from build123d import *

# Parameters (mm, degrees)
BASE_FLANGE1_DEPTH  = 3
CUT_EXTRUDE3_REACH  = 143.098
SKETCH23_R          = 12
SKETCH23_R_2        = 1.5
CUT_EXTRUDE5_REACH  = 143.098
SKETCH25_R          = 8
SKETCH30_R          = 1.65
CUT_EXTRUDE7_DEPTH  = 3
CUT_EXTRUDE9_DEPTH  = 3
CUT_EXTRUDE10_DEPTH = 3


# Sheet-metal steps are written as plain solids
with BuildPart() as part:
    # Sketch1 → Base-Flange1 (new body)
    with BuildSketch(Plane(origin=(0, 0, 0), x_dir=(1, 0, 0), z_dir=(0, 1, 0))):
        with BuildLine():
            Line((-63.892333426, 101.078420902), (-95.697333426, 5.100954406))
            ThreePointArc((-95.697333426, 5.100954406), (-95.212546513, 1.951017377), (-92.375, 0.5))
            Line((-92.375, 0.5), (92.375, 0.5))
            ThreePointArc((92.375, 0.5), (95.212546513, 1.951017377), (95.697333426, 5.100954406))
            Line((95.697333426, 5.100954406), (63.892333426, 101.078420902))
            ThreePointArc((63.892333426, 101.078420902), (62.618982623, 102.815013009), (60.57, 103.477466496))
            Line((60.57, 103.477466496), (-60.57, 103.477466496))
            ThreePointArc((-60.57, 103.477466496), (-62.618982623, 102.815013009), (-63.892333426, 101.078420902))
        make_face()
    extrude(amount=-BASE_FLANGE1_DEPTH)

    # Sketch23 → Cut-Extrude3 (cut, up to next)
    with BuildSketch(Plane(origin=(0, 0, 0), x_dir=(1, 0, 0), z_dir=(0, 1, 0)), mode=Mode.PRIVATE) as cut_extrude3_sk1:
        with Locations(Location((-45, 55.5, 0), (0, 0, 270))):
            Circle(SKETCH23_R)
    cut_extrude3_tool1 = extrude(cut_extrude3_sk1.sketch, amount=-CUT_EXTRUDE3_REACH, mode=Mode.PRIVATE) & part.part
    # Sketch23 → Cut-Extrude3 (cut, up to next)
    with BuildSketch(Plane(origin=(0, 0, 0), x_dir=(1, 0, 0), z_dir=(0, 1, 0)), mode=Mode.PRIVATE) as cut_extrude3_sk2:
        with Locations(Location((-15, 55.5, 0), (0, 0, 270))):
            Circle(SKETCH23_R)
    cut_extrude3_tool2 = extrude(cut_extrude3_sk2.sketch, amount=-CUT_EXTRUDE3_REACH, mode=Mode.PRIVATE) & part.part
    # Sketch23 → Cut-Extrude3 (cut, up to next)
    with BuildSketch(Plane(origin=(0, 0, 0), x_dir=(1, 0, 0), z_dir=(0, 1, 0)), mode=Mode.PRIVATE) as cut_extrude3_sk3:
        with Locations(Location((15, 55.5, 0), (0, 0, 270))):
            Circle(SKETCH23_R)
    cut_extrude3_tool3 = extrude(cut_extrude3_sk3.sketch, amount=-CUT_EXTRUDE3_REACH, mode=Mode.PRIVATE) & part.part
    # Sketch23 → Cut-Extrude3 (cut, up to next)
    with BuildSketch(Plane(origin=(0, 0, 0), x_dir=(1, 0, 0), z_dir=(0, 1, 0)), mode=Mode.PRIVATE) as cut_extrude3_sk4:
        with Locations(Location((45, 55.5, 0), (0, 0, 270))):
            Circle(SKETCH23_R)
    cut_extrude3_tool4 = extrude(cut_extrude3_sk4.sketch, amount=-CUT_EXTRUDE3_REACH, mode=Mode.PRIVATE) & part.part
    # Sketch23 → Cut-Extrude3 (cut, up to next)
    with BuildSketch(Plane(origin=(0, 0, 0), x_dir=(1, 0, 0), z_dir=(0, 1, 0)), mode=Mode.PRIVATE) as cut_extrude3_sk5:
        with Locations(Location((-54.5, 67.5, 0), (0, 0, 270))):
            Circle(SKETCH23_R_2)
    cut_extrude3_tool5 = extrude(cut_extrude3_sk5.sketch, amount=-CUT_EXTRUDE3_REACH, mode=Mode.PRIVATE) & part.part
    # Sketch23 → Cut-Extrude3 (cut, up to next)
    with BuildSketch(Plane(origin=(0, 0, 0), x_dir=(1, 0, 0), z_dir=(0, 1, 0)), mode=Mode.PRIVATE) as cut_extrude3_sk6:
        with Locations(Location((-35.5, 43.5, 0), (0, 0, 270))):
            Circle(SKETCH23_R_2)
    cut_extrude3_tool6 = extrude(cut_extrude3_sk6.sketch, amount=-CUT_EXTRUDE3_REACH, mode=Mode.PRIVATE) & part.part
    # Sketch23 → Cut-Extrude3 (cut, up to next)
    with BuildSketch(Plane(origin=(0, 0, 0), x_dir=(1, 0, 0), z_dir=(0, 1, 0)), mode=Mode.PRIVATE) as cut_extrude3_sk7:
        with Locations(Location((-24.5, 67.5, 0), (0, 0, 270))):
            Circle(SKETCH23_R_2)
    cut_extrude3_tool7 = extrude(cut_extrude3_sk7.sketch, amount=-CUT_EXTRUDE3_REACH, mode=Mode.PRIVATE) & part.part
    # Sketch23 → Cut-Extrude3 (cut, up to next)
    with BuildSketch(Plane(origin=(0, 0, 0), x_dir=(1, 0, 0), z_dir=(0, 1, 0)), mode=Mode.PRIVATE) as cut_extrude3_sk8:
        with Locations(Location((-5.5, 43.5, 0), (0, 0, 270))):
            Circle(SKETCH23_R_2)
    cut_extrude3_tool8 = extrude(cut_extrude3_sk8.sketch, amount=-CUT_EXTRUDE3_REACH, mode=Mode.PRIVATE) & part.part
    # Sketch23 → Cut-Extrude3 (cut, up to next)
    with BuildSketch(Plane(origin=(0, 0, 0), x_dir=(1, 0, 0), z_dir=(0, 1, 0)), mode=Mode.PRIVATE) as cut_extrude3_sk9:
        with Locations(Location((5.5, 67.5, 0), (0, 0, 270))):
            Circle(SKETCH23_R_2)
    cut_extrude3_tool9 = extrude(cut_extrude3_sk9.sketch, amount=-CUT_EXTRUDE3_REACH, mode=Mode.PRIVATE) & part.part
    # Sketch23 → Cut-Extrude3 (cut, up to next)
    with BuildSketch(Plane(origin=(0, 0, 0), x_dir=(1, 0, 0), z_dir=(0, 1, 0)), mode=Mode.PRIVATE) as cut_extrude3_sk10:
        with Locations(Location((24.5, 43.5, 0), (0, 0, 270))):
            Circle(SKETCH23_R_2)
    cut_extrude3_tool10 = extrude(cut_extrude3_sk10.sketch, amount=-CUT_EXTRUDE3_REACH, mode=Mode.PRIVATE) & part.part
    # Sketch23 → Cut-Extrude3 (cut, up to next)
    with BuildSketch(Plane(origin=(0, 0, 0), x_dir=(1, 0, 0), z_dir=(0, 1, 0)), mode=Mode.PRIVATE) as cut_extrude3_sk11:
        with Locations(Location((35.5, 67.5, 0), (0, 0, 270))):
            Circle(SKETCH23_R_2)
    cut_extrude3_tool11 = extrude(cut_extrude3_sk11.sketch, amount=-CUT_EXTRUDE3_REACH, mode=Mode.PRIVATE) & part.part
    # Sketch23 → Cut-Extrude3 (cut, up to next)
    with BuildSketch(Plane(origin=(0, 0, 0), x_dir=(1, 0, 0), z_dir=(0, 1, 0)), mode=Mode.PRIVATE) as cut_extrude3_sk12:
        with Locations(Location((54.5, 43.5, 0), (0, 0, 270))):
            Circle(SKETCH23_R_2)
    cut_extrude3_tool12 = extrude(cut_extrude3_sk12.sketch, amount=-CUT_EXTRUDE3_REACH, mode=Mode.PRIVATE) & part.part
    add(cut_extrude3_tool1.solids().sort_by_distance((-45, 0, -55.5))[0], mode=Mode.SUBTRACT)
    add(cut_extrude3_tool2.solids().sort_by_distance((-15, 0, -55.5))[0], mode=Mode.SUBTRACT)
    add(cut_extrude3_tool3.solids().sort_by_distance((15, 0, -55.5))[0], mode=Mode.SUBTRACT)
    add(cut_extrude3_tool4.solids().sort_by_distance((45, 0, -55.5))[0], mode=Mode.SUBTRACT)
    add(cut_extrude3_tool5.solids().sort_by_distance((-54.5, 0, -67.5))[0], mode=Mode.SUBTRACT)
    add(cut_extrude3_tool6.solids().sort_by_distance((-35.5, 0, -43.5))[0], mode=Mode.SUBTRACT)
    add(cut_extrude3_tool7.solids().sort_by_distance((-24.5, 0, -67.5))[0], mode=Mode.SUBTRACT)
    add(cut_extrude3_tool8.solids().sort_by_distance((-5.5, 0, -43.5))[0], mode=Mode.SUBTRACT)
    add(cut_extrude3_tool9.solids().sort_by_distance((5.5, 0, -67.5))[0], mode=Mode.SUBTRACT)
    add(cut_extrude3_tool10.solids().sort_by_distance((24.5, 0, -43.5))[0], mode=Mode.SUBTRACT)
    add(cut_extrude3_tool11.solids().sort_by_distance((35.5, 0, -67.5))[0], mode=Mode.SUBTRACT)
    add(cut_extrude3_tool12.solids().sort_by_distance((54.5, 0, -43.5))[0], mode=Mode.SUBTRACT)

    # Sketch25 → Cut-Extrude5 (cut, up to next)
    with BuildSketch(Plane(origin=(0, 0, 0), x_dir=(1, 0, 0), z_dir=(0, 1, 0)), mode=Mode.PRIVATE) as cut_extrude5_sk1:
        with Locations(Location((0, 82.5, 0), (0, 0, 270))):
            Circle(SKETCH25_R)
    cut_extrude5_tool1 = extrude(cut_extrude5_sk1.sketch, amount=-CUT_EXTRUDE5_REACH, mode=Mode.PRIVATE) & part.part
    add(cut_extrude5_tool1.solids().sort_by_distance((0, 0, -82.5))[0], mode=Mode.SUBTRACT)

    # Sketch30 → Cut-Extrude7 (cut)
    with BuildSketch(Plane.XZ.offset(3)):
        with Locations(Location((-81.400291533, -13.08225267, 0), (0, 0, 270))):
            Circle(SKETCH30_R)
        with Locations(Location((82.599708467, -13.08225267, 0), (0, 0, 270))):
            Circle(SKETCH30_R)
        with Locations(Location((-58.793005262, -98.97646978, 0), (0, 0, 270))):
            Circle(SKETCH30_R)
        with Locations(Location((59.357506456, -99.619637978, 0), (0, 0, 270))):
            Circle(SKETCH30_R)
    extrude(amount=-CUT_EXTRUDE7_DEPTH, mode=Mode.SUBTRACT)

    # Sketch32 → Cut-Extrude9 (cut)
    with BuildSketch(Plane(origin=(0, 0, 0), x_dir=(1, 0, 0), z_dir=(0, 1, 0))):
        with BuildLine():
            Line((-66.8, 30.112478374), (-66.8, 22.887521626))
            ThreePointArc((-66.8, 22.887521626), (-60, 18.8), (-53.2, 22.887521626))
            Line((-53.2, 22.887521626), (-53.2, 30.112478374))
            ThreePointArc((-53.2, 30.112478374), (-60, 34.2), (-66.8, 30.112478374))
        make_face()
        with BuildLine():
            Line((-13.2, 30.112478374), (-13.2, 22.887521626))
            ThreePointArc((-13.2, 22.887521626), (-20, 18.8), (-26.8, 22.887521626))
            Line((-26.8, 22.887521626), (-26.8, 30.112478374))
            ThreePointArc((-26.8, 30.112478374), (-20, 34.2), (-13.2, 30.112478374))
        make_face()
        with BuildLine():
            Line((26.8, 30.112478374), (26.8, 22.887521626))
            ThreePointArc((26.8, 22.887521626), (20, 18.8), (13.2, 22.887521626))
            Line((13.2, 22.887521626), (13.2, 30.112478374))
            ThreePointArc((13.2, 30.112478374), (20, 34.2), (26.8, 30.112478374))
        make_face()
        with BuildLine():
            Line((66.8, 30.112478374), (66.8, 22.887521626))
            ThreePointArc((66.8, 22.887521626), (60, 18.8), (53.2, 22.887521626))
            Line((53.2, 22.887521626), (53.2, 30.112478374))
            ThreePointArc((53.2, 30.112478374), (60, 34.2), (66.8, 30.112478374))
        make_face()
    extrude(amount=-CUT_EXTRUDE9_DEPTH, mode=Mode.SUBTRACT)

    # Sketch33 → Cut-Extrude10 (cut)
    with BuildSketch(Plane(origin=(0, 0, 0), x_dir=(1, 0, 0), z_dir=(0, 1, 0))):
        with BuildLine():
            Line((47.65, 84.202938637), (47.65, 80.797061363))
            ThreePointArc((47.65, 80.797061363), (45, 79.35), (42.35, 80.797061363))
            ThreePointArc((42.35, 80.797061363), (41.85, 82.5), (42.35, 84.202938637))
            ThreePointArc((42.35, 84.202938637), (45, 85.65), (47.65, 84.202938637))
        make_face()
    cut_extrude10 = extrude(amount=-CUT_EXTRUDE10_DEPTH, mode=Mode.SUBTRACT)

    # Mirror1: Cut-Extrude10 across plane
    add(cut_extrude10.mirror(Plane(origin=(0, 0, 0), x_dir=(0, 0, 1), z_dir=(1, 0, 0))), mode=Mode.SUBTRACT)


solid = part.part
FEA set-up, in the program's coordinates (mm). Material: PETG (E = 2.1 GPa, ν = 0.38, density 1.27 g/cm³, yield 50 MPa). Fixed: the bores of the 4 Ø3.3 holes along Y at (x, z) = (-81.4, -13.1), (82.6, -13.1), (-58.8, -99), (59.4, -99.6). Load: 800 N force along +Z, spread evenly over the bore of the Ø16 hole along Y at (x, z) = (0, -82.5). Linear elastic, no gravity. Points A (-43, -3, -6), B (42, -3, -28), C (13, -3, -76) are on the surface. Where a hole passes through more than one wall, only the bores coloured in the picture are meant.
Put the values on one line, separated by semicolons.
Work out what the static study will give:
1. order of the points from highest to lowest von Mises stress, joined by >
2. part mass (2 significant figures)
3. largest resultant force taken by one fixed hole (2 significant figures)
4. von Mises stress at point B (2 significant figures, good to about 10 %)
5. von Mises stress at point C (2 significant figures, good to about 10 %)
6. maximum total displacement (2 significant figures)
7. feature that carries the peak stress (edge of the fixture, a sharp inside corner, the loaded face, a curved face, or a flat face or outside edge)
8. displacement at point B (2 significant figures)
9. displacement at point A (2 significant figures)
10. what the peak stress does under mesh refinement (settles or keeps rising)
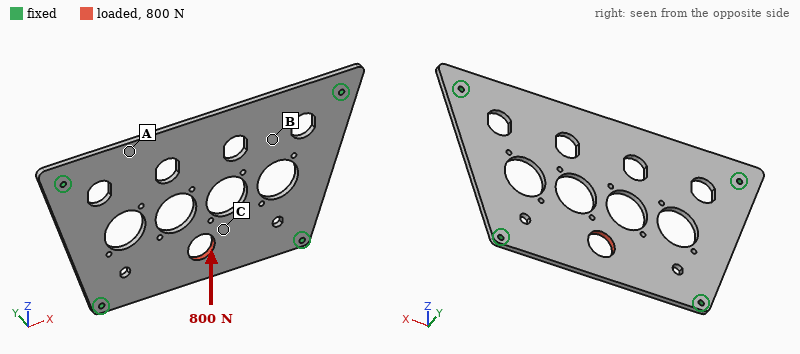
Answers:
C > B > A; 52 g; 310 N; 3.9 MPa; 6.8 MPa; 0.44 mm; edge of the fixture; 0.15 mm; 0.14 mm; keeps rising
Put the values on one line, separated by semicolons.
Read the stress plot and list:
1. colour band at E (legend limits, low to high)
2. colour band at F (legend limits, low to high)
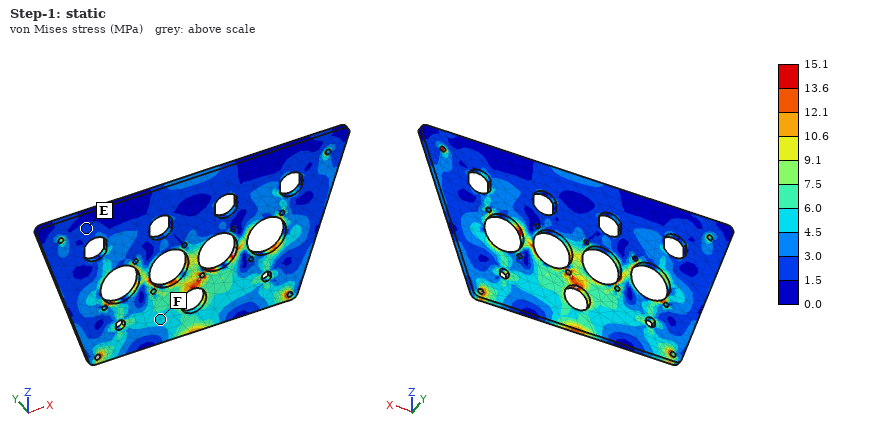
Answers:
1.5 to 3.0 MPa; 4.5 to 6.0 MPa
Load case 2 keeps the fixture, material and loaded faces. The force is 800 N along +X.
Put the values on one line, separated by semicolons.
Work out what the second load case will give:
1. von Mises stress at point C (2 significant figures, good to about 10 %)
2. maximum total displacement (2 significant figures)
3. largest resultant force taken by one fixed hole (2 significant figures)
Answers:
5.2 MPa; 0.17 mm; 330 N
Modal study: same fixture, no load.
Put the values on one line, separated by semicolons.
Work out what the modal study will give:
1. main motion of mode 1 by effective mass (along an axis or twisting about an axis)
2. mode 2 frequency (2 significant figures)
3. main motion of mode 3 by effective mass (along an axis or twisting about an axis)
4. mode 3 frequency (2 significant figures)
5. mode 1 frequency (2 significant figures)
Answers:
along Y; 270 Hz; twisting about Z; 370 Hz; 150 Hz
